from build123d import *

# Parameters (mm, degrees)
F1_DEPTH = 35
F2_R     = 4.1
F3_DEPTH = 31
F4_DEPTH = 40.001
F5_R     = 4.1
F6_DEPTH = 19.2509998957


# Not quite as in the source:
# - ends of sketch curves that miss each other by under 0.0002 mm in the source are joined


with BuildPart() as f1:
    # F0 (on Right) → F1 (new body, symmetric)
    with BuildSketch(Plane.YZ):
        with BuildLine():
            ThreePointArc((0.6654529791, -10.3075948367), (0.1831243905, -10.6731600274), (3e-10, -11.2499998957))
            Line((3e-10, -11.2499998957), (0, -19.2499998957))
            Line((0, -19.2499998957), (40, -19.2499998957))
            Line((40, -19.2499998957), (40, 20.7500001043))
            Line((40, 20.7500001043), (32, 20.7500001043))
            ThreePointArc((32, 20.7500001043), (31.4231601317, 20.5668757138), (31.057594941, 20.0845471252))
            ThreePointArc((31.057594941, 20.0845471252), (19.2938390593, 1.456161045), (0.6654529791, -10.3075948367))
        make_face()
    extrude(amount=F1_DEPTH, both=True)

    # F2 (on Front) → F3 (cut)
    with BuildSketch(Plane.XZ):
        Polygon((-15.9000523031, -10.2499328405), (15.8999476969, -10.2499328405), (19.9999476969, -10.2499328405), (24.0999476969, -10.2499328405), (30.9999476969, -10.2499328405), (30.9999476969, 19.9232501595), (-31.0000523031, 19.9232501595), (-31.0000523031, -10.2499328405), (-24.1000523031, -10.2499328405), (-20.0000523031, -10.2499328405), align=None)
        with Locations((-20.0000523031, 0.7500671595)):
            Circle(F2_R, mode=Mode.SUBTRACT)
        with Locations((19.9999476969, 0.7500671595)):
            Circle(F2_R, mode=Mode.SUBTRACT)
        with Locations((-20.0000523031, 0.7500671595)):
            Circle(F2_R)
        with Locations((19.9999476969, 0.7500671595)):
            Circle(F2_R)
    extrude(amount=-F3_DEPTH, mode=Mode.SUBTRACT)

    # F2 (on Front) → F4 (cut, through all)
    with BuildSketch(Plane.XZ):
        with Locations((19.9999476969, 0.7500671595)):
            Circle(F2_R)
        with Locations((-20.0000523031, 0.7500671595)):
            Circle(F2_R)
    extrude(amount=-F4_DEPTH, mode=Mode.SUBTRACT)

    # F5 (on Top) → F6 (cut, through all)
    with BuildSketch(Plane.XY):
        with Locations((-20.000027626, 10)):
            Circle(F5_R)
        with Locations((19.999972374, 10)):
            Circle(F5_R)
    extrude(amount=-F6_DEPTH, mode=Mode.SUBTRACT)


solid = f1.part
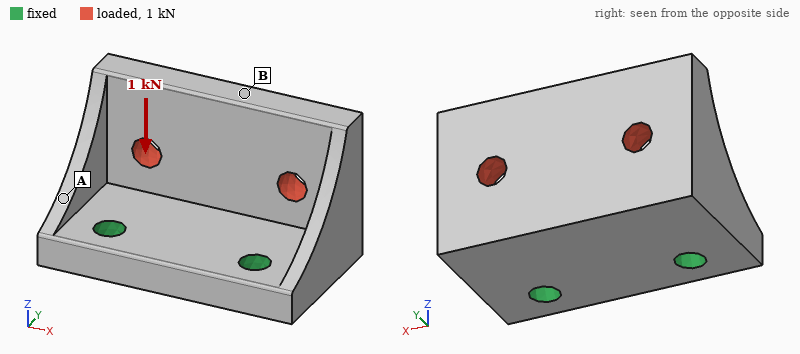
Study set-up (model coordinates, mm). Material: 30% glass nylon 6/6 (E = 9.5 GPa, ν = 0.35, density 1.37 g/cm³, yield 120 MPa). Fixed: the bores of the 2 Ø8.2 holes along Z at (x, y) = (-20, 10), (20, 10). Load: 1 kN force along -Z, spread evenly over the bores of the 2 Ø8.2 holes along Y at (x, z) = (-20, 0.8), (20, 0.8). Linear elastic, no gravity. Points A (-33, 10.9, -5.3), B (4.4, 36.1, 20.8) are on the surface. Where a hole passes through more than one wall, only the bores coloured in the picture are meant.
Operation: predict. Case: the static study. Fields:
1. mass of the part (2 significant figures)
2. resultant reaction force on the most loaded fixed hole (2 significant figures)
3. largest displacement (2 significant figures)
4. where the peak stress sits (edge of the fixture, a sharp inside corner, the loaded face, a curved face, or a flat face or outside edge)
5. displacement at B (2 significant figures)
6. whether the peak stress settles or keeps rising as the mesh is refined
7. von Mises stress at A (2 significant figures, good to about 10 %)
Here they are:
62 g
500 N
0.25 mm
edge of the fixture
0.24 mm
keeps rising
15 MPa
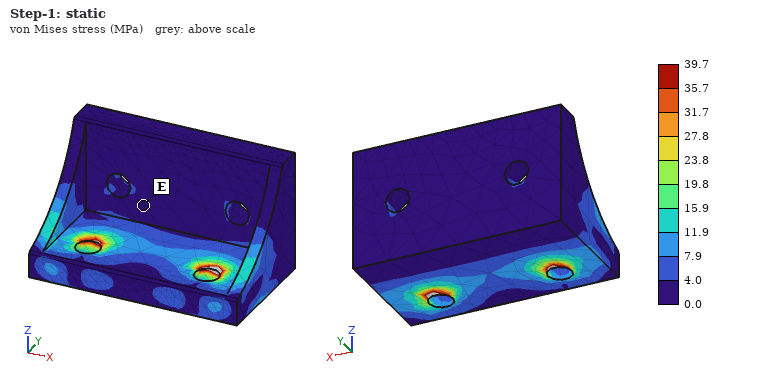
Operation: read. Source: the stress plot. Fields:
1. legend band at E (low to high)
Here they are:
0.0 to 4.0 MPa
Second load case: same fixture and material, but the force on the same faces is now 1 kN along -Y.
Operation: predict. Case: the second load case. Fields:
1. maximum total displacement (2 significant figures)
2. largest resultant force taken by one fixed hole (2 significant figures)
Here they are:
0.25 mm
500 N
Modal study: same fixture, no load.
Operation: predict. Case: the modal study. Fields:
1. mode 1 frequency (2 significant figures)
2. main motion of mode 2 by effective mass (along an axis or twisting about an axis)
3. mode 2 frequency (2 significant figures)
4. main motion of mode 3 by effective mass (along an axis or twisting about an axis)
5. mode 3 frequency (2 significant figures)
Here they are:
1700 Hz
along X
2400 Hz
along Z
4600 Hz
